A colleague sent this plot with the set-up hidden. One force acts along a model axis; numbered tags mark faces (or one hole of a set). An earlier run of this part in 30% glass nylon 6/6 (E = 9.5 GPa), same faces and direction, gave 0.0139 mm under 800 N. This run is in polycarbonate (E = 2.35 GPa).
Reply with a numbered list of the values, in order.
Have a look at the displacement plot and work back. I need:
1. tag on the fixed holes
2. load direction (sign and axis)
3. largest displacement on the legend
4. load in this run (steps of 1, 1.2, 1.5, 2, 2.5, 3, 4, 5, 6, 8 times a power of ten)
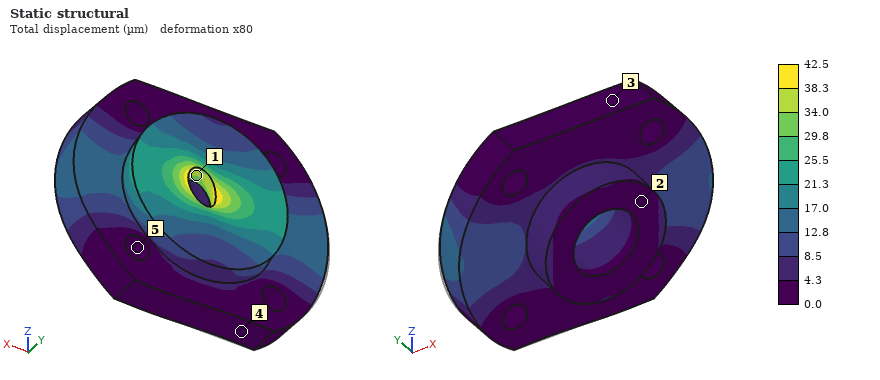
1. 5
2. +X
3. 42.5 µm
4. 600 N
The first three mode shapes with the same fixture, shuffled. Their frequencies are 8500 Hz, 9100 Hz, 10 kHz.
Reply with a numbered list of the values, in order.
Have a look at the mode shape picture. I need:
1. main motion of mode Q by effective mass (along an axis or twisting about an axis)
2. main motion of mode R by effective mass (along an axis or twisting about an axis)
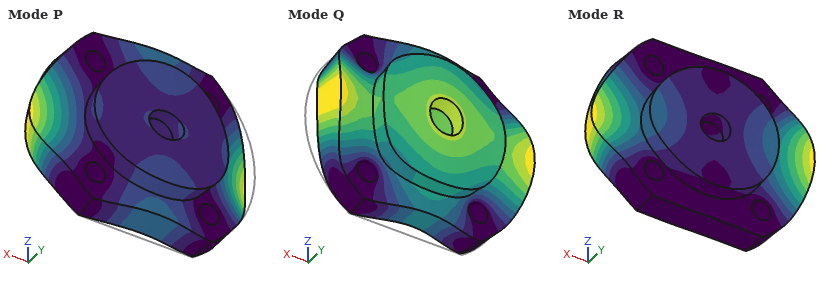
1. along Y
2. twisting about Z
